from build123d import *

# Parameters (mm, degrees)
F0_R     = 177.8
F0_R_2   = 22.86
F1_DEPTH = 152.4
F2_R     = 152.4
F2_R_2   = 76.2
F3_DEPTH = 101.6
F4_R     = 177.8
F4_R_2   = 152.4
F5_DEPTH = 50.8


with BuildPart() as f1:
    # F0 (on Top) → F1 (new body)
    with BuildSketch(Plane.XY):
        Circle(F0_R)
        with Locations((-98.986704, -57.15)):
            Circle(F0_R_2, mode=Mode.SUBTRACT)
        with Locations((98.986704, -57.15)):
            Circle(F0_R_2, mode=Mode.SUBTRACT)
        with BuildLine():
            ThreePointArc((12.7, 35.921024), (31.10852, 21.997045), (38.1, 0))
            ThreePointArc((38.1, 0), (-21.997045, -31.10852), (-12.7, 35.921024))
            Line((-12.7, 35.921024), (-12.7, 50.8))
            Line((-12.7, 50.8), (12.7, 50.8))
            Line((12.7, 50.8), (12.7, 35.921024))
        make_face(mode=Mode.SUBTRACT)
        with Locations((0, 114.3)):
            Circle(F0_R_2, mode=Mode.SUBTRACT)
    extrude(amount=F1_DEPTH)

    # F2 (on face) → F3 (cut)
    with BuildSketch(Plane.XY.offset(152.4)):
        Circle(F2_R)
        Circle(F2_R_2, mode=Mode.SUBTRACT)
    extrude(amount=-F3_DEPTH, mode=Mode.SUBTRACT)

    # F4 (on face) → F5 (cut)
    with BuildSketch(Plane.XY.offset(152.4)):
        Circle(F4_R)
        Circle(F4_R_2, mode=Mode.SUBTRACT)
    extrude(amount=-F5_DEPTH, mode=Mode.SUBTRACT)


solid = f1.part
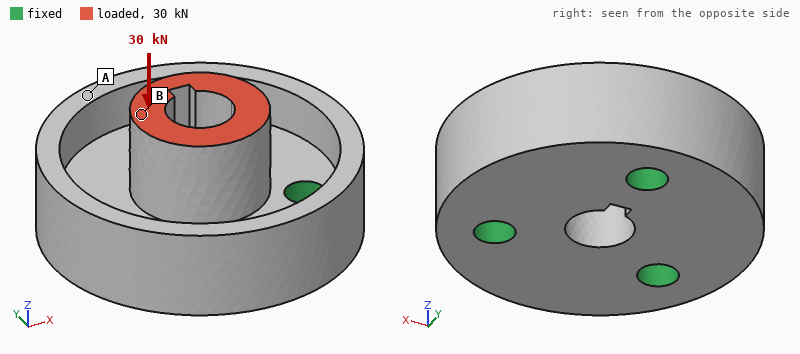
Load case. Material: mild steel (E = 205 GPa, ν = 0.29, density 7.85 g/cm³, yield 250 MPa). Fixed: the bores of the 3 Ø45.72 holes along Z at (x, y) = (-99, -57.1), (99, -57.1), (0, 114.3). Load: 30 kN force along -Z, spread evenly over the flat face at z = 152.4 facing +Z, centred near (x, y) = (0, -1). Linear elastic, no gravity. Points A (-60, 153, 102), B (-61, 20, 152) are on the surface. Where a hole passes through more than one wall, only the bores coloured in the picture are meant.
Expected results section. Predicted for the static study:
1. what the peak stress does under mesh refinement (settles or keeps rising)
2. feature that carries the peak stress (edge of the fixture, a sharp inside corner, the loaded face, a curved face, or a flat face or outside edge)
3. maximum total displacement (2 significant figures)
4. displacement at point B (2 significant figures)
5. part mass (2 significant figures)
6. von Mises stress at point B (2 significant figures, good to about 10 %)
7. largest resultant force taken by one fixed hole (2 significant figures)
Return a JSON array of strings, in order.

["keeps rising", "edge of the fixture", "2.6 µm", "2.5 µm", "57 kg", "2.3 MPa", "10 kN"]
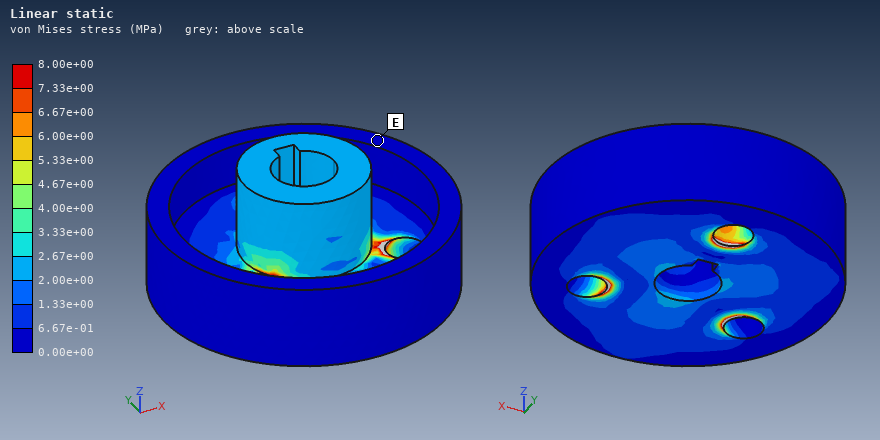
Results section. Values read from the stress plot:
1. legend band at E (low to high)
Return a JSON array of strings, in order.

["0.00e+00 to 6.67e-01 MPa"]
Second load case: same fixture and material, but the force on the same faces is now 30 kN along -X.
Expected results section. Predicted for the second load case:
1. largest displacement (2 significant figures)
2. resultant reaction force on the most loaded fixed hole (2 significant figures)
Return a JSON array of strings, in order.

["16 µm", "22 kN"]
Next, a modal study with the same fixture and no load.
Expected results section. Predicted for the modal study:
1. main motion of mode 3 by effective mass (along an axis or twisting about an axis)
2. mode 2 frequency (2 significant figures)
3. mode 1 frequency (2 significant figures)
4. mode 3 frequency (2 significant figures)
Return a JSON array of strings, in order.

["along Z", "2500 Hz", "2500 Hz", "3200 Hz"]
